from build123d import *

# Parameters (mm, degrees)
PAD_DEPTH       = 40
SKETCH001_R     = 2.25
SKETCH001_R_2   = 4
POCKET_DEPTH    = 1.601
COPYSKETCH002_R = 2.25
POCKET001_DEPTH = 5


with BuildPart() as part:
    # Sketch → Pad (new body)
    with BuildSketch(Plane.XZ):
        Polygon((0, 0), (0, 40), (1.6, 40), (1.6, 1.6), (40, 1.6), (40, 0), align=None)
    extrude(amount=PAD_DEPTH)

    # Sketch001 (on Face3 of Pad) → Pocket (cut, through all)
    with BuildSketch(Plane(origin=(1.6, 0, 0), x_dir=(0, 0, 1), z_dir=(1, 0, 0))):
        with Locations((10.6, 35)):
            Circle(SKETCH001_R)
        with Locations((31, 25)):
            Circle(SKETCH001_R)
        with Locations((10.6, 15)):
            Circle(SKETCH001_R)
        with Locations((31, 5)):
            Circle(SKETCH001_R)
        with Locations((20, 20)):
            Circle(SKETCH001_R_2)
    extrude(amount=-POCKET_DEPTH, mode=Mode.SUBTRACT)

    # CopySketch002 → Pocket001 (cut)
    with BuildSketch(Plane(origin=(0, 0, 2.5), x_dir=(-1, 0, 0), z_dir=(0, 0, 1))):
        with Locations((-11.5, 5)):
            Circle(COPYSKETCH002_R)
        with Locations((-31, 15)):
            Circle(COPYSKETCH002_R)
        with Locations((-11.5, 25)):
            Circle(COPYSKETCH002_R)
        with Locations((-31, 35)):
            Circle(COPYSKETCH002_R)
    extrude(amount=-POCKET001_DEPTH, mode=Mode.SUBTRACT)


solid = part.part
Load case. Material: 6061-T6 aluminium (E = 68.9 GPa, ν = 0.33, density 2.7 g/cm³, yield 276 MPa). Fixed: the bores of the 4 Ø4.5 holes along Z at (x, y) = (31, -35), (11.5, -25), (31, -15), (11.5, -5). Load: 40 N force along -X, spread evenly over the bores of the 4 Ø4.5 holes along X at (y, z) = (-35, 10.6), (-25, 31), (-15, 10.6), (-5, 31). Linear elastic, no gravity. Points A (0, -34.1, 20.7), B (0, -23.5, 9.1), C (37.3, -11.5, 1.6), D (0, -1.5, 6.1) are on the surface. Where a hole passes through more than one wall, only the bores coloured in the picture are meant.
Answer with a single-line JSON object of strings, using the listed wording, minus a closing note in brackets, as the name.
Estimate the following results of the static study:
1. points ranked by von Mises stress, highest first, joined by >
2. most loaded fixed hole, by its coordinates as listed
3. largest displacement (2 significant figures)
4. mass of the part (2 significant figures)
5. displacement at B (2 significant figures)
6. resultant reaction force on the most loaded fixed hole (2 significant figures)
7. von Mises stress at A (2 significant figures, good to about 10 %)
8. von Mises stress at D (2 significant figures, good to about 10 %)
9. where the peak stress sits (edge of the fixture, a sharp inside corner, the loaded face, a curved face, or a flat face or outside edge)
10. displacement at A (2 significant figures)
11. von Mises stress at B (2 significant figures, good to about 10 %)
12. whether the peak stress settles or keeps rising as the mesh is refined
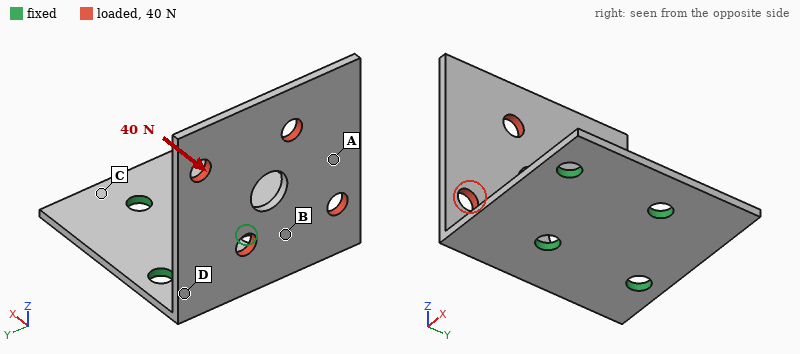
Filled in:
{"points ranked by von Mises stress, highest first, joined by >": "D > B > A > C", "most loaded fixed hole, by its coordinates as listed": "(11.5, -25)", "largest displacement": "0.65 mm", "mass of the part": "13 g", "displacement at B": "0.100 mm", "resultant reaction force on the most loaded fixed hole": "24 N", "von Mises stress at A": "14 MPa", "von Mises stress at D": "40 MPa", "where the peak stress sits": "edge of the fixture", "displacement at A": "0.26 mm", "von Mises stress at B": "28 MPa", "whether the peak stress settles or keeps rising as the mesh is refined": "keeps rising"}
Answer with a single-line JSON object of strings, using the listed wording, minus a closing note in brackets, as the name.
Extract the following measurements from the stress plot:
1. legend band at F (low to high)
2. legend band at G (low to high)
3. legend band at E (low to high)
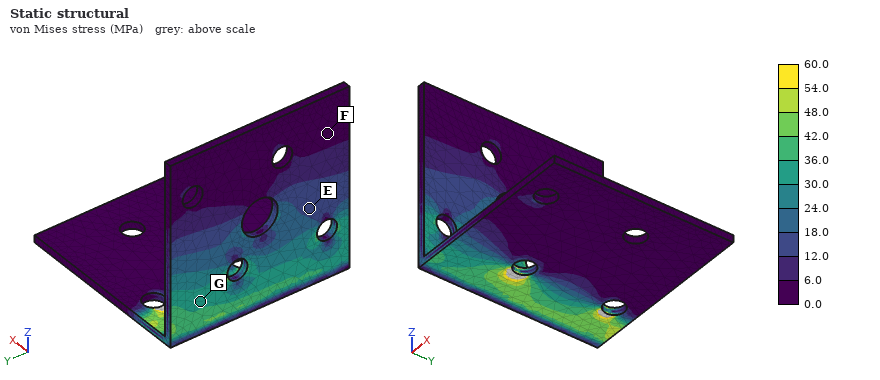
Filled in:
{"legend band at F": "0.0 to 6.0 MPa", "legend band at G": "30.0 to 36.0 MPa", "legend band at E": "12.0 to 18.0 MPa"}
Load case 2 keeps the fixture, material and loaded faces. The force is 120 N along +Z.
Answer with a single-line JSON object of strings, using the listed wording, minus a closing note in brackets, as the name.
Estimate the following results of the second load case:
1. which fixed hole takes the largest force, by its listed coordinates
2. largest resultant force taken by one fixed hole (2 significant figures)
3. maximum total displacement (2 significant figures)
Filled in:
{"which fixed hole takes the largest force, by its listed coordinates": "(11.5, -25)", "largest resultant force taken by one fixed hole": "92 N", "maximum total displacement": "0.25 mm"}
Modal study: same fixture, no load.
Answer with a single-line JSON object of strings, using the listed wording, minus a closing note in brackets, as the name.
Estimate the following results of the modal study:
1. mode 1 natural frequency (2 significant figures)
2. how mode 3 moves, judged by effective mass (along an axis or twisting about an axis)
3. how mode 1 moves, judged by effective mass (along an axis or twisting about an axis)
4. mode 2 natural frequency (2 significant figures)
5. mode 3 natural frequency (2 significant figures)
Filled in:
{"mode 1 natural frequency": "620 Hz", "how mode 3 moves, judged by effective mass": "along Y", "how mode 1 moves, judged by effective mass": "along X", "mode 2 natural frequency": "1600 Hz", "mode 3 natural frequency": "2200 Hz"}
